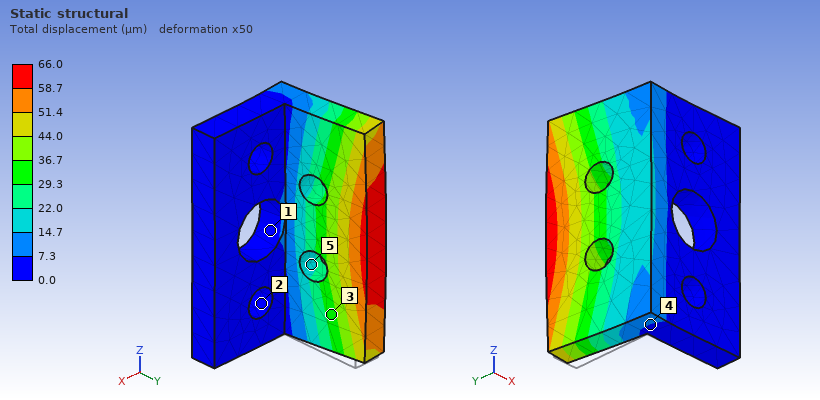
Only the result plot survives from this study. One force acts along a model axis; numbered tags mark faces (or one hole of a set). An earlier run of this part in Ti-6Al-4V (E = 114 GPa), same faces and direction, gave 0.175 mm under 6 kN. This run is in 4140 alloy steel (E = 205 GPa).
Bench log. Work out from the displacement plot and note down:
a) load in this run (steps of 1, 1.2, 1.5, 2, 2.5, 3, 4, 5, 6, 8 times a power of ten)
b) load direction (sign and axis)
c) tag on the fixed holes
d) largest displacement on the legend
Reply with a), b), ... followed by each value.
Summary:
a) 4 kN
b) -X
c) 2
d) 66.0 µm
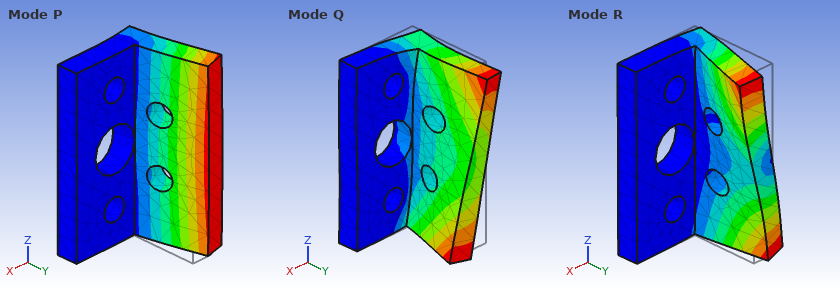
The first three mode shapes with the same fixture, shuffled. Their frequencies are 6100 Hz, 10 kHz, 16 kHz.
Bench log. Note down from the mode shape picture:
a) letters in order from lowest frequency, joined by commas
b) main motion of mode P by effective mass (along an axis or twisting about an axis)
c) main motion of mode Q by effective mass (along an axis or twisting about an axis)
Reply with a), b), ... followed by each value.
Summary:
a) P, R, Q
b) along X
c) along Z
